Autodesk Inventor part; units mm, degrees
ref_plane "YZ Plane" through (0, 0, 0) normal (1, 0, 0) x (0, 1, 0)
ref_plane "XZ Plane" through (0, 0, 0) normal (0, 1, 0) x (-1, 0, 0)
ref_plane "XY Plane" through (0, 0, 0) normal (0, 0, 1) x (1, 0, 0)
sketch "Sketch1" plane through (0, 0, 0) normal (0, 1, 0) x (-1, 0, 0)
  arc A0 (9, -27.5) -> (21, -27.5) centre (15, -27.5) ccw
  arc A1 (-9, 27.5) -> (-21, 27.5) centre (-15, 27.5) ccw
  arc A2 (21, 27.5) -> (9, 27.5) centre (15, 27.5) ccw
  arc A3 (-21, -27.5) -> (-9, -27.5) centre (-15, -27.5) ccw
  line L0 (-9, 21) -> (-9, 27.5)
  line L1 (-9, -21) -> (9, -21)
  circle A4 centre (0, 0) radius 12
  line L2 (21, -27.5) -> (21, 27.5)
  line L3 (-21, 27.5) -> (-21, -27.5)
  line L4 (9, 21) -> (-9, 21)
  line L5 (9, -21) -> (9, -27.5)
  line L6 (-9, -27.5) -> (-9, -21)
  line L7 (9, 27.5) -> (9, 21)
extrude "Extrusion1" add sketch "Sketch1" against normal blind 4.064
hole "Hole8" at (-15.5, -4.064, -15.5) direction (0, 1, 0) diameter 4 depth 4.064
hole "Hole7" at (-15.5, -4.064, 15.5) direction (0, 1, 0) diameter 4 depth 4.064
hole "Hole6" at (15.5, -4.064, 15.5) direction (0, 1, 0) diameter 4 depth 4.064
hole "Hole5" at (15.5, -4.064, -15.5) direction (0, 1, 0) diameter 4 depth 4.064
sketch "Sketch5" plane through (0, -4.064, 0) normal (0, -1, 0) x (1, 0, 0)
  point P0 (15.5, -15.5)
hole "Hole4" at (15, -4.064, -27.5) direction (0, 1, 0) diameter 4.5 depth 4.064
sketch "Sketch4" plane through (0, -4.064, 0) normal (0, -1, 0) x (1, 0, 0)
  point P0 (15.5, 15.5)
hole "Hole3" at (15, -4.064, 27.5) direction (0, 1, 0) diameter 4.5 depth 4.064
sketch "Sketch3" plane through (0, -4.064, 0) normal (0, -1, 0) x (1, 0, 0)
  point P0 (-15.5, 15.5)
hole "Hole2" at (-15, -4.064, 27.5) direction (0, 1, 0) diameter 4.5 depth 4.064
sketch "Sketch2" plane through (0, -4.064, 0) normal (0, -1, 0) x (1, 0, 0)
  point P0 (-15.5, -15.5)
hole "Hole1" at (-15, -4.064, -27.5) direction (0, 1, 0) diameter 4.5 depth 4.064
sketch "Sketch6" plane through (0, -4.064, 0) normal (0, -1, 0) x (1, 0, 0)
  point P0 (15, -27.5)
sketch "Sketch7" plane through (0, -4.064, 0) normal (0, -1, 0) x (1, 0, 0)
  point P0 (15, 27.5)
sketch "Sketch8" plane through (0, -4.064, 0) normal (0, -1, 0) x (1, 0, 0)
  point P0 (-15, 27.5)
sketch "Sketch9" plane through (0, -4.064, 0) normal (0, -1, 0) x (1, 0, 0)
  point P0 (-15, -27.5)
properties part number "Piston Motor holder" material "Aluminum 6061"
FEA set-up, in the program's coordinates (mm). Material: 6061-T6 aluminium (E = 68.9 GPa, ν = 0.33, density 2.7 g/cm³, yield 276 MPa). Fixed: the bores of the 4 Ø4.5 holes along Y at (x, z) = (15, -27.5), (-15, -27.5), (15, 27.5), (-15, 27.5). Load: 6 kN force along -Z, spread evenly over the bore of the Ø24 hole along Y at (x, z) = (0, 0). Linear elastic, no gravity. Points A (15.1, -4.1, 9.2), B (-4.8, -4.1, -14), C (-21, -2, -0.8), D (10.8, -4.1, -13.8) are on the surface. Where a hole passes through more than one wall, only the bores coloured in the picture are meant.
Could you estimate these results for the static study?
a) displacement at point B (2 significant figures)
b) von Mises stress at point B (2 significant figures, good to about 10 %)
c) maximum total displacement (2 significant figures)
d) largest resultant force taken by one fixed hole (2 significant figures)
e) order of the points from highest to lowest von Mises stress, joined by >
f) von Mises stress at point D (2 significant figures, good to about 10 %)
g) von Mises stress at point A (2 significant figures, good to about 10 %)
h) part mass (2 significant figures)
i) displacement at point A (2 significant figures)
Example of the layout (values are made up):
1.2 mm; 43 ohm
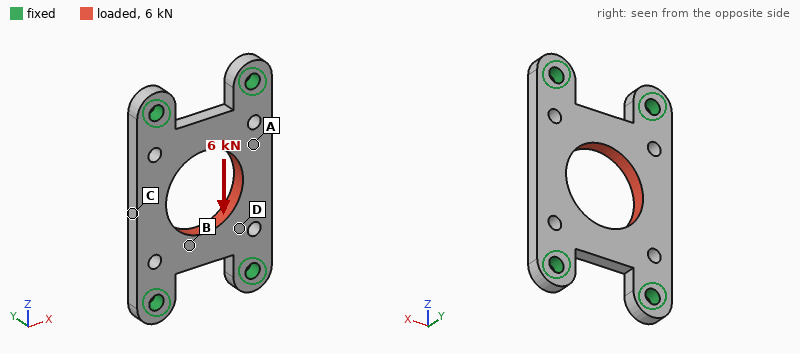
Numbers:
11 µm; 25 MPa; 13 µm; 1.6 kN; D > B > A > C; 34 MPa; 15 MPa; 19 g; 7.6 µm
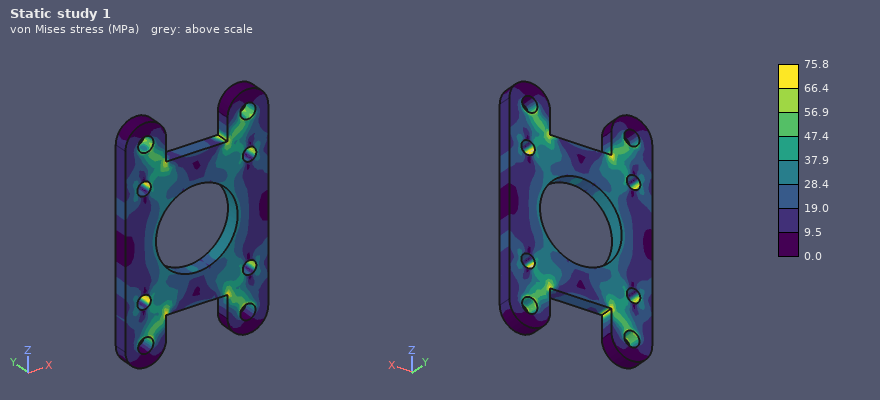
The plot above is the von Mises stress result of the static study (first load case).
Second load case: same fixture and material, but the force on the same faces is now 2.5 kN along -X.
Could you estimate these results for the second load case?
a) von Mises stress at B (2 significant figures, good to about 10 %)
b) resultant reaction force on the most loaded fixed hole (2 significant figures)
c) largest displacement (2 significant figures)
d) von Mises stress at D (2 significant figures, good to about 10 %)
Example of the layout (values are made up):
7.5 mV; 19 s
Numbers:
25 MPa; 680 N; 18 µm; 10 MPa
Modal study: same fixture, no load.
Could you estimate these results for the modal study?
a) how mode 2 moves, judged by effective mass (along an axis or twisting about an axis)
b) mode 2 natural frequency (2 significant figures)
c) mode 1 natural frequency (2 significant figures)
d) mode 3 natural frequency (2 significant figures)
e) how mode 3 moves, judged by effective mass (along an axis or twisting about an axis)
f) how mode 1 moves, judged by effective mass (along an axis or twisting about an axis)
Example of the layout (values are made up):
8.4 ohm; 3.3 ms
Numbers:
twisting about Z; 8600 Hz; 7000 Hz; 14 kHz; twisting about X; along Y
